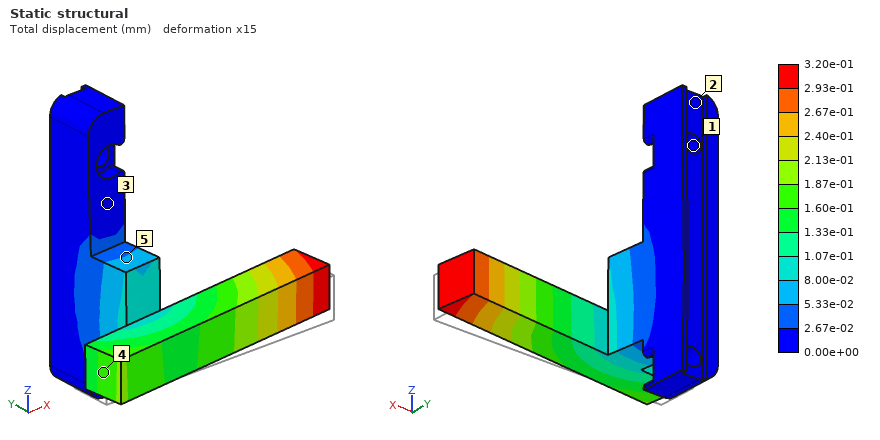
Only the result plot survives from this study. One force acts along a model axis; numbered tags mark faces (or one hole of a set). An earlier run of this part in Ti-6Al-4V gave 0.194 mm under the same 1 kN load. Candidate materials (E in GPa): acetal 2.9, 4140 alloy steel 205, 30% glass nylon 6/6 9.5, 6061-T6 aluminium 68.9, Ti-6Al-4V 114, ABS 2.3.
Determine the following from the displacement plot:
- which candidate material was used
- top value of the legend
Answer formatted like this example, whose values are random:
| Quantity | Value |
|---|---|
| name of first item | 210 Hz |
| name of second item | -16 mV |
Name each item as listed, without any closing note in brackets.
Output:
| Quantity | Value |
|---|---|
| which candidate material was used | 6061-T6 aluminium |
| top value of the legend | 3.20e-01 mm |
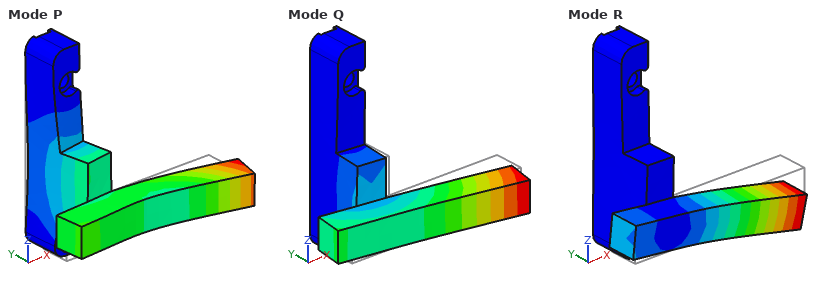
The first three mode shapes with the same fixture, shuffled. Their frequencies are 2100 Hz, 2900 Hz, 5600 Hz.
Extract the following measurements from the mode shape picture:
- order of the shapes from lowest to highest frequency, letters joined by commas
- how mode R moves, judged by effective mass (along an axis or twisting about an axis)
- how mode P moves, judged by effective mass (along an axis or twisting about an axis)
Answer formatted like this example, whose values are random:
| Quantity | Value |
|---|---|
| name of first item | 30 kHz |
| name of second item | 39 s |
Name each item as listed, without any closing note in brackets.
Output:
| Quantity | Value |
|---|---|
| order of the shapes from lowest to highest frequency, letters joined by commas | Q, R, P |
| how mode R moves, judged by effective mass | along Z |
| how mode P moves, judged by effective mass | along X |
